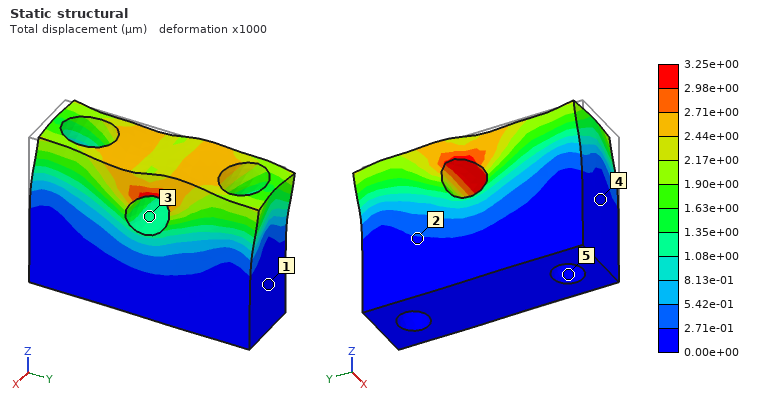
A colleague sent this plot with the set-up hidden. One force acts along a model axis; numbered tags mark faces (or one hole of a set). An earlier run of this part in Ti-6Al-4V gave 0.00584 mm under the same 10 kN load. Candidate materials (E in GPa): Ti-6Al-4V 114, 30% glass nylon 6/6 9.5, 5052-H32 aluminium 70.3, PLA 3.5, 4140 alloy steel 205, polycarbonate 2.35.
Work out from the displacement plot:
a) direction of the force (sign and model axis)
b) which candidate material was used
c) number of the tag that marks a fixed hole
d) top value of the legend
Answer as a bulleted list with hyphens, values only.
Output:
- +Y
- 4140 alloy steel
- 5
- 3.25e+00 µm
